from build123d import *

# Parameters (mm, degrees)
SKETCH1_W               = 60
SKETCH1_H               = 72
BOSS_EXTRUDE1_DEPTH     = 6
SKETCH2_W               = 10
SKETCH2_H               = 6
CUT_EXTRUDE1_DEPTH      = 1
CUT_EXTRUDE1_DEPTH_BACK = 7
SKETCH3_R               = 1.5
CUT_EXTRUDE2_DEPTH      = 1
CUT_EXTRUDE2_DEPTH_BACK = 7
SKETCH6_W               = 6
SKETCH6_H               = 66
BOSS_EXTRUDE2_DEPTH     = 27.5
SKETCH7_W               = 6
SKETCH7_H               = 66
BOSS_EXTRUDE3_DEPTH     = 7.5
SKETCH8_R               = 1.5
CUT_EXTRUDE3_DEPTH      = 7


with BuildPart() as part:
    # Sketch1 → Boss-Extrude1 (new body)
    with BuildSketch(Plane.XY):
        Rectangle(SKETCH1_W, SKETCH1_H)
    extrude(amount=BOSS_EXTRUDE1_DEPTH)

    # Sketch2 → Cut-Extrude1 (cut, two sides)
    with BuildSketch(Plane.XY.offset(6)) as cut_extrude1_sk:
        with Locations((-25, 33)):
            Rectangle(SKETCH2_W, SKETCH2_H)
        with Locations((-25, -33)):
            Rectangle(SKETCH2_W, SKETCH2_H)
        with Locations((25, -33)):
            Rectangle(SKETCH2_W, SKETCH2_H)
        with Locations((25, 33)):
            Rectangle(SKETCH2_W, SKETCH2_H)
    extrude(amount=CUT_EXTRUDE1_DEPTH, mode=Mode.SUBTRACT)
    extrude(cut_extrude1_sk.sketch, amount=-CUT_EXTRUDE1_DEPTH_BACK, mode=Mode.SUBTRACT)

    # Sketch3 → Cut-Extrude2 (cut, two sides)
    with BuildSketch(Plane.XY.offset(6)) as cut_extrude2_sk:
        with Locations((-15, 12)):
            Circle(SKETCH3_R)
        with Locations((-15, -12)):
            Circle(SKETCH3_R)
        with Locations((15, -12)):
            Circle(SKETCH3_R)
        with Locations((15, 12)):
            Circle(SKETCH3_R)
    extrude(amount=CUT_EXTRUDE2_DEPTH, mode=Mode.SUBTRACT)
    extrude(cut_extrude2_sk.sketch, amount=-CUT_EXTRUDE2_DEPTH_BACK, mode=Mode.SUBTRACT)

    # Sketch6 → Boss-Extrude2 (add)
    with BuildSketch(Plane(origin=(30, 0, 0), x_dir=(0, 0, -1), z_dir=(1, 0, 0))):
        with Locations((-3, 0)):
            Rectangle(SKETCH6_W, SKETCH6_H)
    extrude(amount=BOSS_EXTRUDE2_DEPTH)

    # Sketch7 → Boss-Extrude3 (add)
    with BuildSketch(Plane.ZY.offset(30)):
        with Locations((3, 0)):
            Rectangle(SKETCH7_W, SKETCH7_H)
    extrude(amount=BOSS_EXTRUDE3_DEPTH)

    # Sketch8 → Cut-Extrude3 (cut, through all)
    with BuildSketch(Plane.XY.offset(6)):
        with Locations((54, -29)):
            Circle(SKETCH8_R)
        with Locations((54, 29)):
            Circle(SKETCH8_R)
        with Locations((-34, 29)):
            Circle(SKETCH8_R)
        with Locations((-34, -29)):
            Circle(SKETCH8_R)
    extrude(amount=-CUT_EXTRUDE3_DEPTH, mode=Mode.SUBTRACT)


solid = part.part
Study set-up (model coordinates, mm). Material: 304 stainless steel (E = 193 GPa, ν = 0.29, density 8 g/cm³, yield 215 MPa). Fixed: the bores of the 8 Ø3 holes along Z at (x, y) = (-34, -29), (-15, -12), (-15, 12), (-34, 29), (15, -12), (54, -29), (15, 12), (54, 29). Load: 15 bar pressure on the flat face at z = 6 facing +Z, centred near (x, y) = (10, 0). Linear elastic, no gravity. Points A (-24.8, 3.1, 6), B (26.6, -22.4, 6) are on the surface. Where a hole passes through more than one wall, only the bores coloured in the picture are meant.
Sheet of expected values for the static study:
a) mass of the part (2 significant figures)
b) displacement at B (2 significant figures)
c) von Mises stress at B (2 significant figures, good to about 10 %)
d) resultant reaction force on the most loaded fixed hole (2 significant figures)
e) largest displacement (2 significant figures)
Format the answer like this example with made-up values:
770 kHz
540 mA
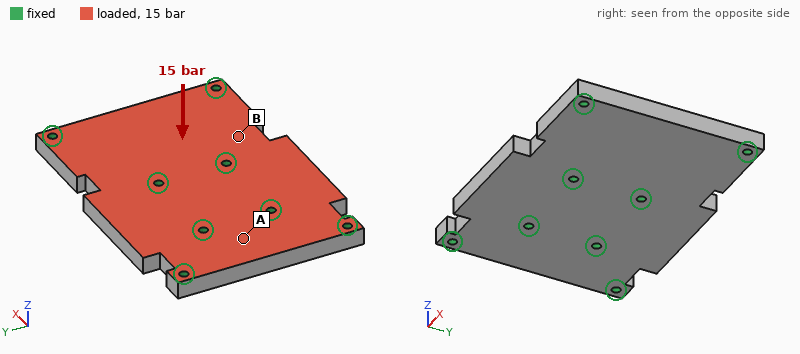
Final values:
300 g
7.9 µm
33 MPa
1.9 kN
17 µm
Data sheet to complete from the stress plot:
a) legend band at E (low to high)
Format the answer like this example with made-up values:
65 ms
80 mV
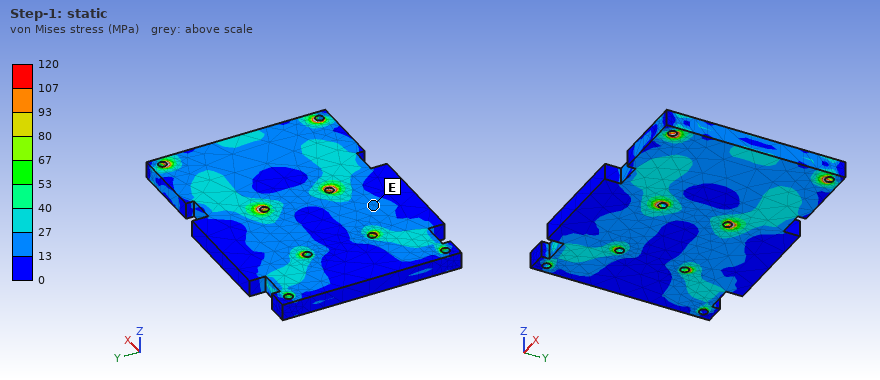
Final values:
13 to 27 MPa
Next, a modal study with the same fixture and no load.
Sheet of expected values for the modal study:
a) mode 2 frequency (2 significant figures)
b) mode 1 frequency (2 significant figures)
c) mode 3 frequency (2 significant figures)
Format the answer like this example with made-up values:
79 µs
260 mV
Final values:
8500 Hz
8000 Hz
8800 Hz
